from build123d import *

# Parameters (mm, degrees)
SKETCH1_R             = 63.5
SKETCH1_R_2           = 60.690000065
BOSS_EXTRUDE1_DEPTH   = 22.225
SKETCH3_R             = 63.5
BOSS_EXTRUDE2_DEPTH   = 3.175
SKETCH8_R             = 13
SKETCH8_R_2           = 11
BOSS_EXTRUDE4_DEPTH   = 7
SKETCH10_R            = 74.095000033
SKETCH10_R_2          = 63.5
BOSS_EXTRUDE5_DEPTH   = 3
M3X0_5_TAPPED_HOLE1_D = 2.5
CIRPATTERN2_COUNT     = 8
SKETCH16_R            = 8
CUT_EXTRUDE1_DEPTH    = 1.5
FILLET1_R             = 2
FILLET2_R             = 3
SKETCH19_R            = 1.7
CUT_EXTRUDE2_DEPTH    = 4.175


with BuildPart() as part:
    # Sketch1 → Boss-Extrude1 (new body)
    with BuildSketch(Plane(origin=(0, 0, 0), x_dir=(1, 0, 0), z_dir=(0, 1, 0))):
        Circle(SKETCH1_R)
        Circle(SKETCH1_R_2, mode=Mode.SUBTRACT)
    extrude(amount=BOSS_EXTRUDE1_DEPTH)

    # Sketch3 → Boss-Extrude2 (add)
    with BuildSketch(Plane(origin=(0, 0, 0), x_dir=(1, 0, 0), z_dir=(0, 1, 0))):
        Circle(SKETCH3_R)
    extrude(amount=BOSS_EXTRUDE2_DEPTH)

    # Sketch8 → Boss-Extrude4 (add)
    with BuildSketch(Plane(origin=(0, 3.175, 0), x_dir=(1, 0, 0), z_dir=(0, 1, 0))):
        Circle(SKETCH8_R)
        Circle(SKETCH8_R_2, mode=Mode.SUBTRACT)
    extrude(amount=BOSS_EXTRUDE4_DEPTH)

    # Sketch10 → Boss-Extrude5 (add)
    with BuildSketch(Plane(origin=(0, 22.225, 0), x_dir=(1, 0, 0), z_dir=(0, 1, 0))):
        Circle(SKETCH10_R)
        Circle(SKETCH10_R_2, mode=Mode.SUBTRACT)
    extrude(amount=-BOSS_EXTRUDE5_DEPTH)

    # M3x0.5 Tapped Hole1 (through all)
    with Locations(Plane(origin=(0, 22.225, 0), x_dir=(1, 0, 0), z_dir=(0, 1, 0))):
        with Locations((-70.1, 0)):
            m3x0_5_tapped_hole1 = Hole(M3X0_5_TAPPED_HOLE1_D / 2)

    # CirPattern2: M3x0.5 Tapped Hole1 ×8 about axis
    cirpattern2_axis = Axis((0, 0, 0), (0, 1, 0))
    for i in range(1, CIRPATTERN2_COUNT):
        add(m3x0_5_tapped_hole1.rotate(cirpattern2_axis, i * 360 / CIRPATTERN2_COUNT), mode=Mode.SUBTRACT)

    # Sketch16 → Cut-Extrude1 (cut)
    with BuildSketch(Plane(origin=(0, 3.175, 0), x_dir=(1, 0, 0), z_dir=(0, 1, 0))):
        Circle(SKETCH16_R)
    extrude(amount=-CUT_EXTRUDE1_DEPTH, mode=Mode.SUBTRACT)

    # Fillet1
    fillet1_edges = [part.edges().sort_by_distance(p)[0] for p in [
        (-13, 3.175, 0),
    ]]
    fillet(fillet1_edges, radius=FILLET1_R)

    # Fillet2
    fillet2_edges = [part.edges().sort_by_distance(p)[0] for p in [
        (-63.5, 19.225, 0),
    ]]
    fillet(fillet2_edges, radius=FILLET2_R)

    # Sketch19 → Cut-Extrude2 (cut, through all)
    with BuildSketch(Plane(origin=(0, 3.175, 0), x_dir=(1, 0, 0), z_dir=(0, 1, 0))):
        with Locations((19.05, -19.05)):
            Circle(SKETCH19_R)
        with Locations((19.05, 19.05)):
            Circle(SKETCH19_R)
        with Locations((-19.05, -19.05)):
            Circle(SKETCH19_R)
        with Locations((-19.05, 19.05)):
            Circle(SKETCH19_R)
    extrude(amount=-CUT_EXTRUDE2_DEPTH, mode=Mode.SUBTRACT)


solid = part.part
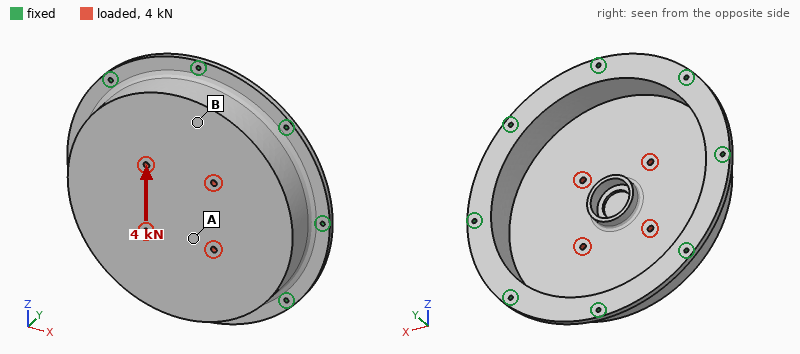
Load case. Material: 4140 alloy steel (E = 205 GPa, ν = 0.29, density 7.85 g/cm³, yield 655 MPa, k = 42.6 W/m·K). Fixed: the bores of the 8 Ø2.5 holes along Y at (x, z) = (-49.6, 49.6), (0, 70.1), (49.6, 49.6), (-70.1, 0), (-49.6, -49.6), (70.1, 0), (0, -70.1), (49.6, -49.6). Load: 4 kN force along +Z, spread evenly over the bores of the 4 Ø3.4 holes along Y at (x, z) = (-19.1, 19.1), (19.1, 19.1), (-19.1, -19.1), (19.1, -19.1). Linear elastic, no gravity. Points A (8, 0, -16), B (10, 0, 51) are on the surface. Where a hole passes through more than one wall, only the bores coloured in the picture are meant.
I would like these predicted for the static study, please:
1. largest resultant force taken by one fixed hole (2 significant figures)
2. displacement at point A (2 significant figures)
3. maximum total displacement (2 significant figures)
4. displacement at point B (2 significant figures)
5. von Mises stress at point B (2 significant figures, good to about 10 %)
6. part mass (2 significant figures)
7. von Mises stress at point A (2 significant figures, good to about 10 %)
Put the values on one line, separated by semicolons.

740 N; 7.7 µm; 9.0 µm; 7.2 µm; 12 MPa; 600 g; 5.1 MPa
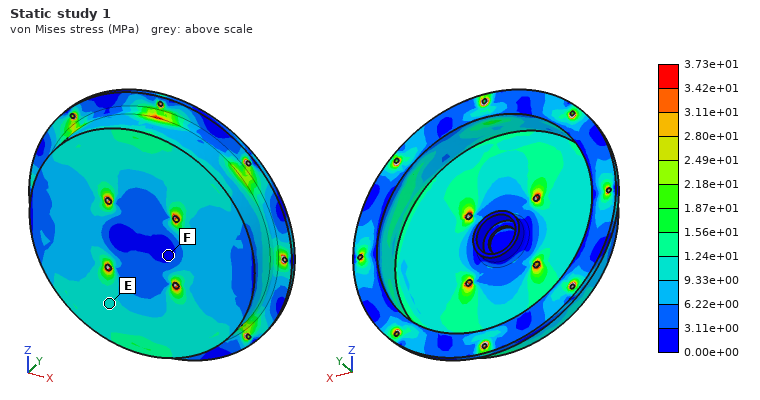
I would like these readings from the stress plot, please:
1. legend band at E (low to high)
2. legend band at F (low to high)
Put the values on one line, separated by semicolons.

9.33e+00 to 1.24e+01 MPa; 0.00e+00 to 3.11e+00 MPa
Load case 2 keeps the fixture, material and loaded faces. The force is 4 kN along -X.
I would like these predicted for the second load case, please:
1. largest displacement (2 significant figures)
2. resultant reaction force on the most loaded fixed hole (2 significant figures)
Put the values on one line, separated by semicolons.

9.0 µm; 740 N
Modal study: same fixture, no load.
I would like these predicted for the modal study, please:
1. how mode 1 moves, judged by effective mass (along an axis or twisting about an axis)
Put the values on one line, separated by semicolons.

along Y
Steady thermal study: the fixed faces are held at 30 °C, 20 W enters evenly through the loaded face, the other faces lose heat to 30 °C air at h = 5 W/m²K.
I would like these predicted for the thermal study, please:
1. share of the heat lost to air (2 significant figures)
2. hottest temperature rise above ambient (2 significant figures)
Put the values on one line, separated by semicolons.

20 %; 41 K
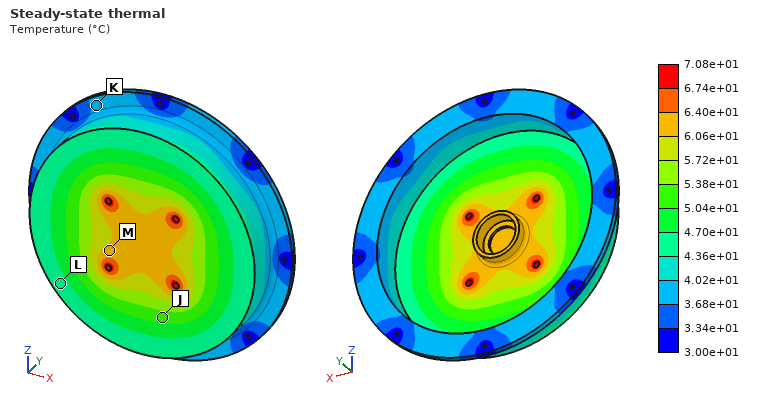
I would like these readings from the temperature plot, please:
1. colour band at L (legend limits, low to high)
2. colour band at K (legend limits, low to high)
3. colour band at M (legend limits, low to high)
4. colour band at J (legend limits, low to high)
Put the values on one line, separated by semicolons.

4.36e+01 to 4.70e+01 °C; 3.68e+01 to 4.02e+01 °C; 6.06e+01 to 6.40e+01 °C; 5.04e+01 to 5.38e+01 °C
